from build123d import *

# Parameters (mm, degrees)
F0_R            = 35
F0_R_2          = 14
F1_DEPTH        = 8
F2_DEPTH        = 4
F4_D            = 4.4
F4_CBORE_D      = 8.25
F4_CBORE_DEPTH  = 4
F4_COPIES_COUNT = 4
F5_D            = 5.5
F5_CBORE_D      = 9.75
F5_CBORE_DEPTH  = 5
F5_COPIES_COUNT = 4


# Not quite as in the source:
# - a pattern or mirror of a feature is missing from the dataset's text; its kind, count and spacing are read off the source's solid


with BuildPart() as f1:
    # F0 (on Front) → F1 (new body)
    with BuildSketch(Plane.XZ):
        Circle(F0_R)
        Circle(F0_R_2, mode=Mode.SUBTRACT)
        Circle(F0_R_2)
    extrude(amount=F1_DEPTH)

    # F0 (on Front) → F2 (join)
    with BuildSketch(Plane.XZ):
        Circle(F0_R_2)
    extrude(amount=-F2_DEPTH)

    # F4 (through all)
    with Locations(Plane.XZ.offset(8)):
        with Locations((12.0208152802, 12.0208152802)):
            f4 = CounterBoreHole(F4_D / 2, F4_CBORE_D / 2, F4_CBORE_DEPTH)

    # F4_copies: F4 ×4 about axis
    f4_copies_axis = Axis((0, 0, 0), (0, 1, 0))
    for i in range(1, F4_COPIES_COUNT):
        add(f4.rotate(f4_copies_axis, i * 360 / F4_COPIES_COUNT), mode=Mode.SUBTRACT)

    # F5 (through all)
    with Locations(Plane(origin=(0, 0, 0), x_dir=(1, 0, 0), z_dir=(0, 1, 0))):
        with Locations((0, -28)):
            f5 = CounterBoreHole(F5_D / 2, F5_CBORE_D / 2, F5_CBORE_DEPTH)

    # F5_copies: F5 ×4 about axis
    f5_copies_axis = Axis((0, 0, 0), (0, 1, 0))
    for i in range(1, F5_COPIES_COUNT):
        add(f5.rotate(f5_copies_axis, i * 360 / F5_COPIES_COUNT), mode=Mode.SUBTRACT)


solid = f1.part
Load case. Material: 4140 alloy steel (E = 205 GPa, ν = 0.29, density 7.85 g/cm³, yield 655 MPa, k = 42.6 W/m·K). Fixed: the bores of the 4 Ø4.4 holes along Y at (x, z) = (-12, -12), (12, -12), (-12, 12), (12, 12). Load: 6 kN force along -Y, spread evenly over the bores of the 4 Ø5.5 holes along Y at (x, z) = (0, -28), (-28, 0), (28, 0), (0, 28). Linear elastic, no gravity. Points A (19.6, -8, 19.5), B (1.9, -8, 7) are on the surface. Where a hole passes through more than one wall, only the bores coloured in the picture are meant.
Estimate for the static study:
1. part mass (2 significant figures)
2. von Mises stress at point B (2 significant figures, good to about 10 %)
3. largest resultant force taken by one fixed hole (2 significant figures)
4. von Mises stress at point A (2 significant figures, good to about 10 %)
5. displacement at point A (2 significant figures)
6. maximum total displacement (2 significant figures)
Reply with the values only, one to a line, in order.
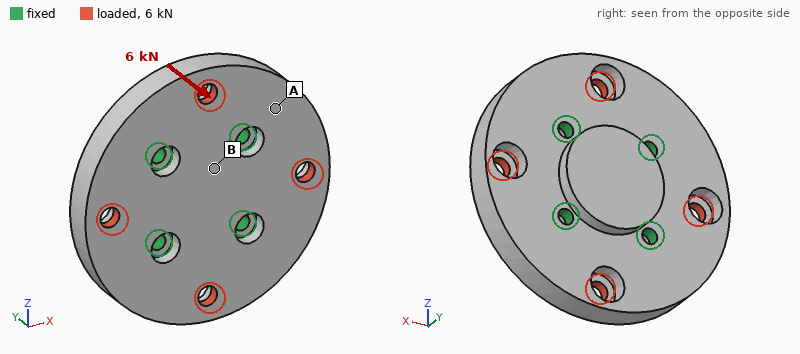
240 g
21 MPa
1.6 kN
41 MPa
4.6 µm
14 µm
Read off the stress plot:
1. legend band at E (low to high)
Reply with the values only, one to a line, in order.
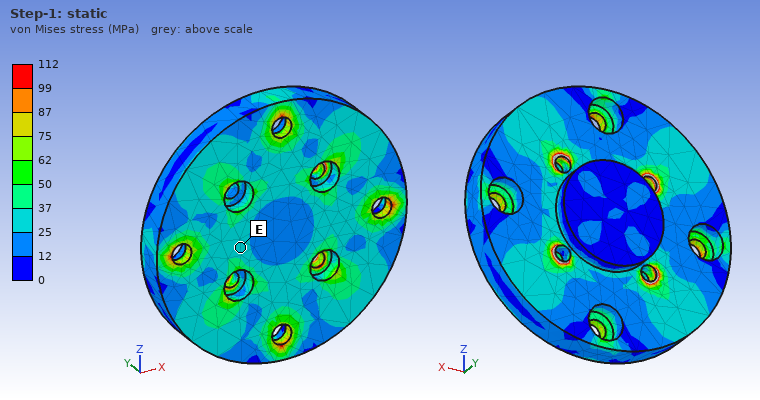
25 to 37 MPa
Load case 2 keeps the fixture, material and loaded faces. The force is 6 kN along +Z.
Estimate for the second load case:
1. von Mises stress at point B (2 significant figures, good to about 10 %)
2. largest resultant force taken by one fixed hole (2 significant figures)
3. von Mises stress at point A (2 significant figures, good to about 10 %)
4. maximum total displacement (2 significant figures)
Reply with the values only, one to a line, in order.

8.5 MPa
1.6 kN
6.4 MPa
6.8 µm
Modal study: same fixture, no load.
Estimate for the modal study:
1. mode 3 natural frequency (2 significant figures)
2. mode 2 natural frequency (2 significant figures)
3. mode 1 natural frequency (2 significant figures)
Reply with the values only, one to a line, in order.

11 kHz
11 kHz
11 kHz
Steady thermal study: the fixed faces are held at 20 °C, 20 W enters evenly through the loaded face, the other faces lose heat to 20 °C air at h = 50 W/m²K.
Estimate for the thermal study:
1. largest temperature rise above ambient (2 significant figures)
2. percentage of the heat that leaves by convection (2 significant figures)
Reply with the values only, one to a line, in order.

16 K
17 %
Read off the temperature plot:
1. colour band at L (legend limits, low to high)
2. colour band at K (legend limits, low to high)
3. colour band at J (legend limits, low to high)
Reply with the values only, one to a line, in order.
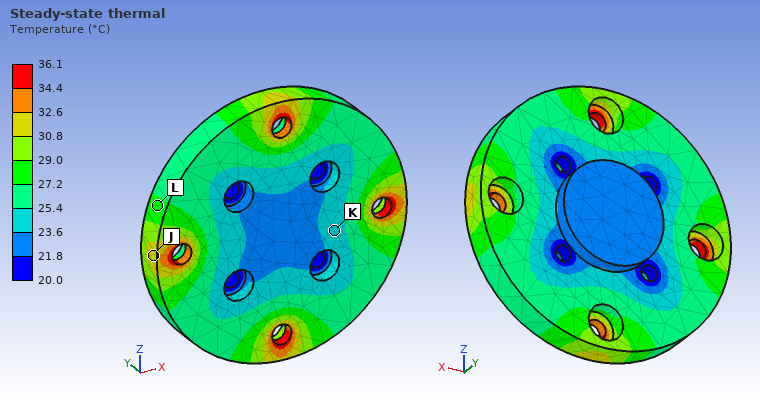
27.2 to 29.0 °C
23.6 to 25.4 °C
30.8 to 32.6 °C
